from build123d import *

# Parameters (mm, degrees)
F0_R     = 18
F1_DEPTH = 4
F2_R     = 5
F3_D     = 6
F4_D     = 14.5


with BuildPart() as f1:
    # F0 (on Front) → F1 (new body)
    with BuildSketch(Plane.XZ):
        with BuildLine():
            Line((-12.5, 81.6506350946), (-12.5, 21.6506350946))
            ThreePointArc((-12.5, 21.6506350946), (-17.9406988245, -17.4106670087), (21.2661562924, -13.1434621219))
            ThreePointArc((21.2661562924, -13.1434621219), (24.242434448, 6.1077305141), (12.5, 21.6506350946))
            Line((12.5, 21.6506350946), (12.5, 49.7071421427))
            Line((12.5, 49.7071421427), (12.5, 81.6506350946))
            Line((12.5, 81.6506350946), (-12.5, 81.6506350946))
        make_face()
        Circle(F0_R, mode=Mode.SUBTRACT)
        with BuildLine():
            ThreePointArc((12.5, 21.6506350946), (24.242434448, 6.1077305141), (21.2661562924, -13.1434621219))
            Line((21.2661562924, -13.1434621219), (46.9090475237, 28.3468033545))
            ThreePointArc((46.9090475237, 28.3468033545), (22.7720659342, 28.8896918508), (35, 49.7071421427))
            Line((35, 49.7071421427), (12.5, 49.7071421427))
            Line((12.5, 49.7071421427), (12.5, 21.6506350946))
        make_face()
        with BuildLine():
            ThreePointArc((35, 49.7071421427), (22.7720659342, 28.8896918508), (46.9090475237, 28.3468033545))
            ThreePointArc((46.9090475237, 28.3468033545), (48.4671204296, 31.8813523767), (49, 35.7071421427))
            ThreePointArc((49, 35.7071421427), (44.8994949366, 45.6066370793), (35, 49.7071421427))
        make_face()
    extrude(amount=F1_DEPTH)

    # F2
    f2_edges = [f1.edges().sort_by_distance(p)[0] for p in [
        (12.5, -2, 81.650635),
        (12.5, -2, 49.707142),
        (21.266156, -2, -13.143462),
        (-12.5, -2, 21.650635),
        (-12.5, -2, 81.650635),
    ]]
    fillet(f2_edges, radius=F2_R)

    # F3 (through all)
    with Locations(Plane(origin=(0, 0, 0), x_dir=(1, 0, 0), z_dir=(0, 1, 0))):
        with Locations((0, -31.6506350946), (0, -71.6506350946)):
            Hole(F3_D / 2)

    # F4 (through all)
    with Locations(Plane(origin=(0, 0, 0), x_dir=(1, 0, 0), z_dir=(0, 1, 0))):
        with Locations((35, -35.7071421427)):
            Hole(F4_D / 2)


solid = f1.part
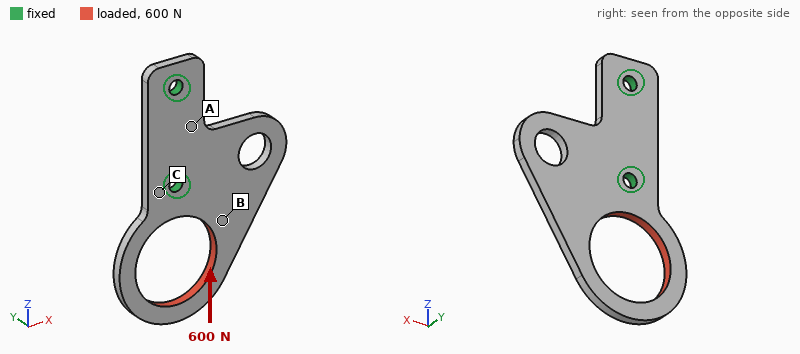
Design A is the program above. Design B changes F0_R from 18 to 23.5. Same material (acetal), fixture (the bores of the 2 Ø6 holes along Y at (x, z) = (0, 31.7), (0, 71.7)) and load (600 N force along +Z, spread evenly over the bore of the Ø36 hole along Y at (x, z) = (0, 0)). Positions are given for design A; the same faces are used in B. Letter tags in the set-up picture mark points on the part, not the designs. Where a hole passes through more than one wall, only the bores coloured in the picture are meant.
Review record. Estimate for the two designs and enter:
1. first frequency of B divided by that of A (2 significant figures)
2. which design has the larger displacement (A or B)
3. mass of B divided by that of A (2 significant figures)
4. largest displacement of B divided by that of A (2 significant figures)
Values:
1.0
B
0.79
65
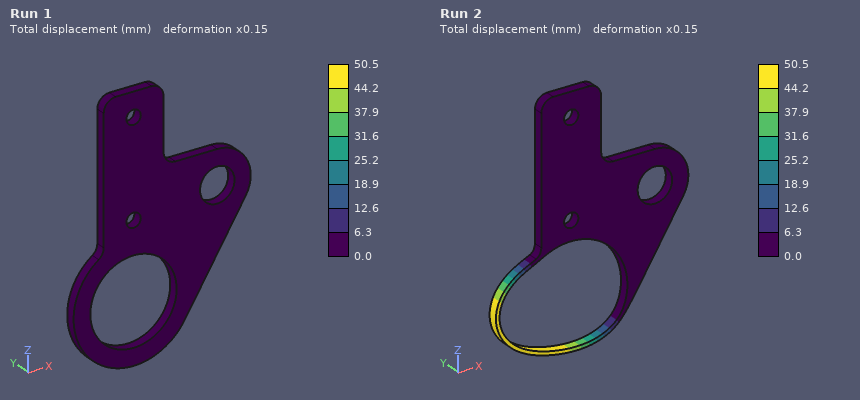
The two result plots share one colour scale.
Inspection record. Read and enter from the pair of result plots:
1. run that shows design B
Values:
Run 2
